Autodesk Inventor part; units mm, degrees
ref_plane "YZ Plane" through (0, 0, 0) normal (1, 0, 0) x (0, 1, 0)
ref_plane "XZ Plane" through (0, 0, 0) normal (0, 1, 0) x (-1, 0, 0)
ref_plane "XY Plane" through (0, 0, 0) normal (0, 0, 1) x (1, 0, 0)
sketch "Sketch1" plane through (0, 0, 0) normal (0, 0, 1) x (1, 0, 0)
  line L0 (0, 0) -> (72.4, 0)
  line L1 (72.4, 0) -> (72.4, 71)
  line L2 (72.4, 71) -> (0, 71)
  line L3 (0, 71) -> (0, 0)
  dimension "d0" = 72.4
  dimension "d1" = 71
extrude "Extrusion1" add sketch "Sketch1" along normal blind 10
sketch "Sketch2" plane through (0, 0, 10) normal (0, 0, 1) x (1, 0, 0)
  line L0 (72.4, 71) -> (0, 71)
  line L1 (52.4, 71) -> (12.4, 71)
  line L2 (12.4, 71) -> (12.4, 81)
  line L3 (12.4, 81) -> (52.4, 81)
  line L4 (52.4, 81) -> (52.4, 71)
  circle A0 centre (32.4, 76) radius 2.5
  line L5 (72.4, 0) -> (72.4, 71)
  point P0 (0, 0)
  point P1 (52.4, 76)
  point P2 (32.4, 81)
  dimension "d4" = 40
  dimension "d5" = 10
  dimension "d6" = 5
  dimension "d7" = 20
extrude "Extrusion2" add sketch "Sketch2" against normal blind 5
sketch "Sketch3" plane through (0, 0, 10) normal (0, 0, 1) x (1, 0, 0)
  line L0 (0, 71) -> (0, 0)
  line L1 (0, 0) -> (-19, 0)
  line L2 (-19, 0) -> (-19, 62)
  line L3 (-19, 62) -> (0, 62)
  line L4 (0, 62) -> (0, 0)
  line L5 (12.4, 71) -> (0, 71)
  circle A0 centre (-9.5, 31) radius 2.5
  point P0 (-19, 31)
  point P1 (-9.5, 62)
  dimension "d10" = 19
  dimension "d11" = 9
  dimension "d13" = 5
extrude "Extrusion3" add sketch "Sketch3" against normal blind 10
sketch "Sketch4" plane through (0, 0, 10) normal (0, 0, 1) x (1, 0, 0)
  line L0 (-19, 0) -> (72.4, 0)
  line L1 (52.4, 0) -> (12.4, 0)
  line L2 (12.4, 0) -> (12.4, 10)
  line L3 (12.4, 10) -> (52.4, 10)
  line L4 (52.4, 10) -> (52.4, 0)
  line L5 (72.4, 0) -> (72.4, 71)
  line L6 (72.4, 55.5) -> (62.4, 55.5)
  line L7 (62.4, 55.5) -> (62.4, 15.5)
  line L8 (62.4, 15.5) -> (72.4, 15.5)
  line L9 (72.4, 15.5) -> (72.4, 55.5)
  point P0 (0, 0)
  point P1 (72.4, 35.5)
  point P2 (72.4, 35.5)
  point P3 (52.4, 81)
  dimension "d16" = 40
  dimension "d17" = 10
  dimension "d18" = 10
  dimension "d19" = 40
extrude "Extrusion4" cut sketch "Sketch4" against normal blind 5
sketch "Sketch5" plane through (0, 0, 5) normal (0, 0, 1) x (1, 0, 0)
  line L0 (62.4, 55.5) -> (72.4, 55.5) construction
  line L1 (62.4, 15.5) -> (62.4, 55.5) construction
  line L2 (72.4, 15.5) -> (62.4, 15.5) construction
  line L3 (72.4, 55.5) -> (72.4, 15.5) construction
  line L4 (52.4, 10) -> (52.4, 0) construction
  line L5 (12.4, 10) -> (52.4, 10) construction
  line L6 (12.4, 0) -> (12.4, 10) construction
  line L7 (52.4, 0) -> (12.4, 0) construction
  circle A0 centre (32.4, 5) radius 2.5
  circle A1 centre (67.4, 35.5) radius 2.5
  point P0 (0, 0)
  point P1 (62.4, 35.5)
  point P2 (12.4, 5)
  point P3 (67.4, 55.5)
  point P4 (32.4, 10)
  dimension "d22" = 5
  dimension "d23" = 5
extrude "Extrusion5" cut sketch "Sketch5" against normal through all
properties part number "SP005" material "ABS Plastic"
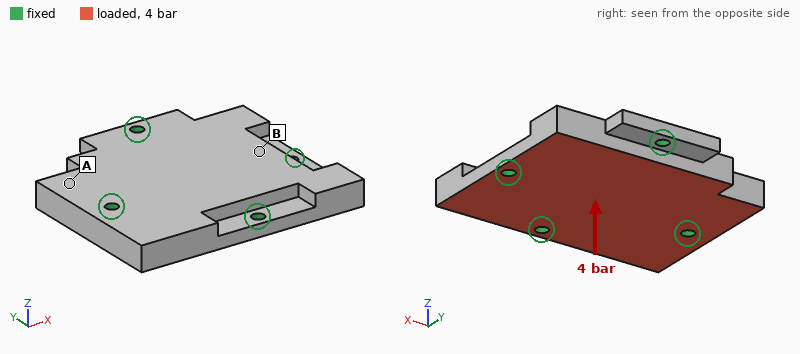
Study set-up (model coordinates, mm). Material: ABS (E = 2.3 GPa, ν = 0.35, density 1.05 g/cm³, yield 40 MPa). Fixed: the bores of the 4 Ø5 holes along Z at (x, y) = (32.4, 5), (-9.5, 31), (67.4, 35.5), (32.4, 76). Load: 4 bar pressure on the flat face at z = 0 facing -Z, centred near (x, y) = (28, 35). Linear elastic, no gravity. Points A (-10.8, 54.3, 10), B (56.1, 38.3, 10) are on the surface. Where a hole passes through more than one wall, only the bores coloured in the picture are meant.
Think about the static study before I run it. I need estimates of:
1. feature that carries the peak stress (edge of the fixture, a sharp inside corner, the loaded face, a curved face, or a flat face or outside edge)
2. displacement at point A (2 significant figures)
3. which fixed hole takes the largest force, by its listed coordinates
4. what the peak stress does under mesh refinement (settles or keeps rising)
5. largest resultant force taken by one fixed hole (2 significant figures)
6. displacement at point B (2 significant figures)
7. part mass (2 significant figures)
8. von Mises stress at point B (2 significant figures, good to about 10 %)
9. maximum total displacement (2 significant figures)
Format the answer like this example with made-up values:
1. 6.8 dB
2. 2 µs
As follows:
1. edge of the fixture
2. 0.15 mm
3. (-9.5, 31)
4. keeps rising
5. 850 N
6. 0.13 mm
7. 64 g
8. 6.3 MPa
9. 0.32 mm
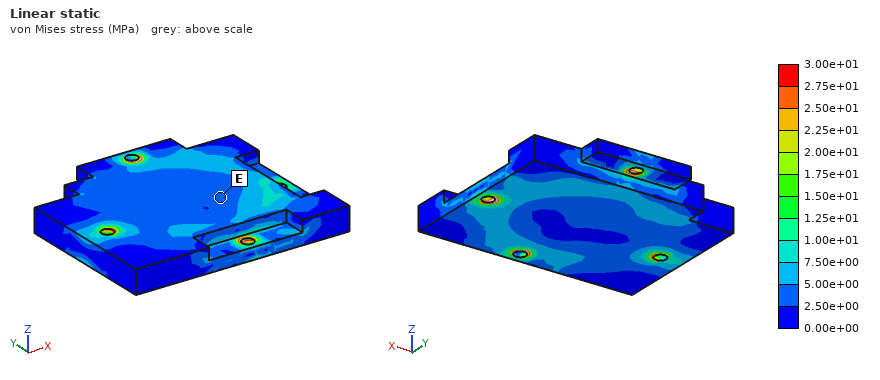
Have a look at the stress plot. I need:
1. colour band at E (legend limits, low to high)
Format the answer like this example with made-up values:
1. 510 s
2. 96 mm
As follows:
1. 2.50e+00 to 5.00e+00 MPa
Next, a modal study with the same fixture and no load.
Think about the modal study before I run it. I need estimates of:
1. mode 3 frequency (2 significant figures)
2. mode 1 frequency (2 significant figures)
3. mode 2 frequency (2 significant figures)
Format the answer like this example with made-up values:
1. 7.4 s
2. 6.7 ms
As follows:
1. 2300 Hz
2. 2000 Hz
3. 2200 Hz
